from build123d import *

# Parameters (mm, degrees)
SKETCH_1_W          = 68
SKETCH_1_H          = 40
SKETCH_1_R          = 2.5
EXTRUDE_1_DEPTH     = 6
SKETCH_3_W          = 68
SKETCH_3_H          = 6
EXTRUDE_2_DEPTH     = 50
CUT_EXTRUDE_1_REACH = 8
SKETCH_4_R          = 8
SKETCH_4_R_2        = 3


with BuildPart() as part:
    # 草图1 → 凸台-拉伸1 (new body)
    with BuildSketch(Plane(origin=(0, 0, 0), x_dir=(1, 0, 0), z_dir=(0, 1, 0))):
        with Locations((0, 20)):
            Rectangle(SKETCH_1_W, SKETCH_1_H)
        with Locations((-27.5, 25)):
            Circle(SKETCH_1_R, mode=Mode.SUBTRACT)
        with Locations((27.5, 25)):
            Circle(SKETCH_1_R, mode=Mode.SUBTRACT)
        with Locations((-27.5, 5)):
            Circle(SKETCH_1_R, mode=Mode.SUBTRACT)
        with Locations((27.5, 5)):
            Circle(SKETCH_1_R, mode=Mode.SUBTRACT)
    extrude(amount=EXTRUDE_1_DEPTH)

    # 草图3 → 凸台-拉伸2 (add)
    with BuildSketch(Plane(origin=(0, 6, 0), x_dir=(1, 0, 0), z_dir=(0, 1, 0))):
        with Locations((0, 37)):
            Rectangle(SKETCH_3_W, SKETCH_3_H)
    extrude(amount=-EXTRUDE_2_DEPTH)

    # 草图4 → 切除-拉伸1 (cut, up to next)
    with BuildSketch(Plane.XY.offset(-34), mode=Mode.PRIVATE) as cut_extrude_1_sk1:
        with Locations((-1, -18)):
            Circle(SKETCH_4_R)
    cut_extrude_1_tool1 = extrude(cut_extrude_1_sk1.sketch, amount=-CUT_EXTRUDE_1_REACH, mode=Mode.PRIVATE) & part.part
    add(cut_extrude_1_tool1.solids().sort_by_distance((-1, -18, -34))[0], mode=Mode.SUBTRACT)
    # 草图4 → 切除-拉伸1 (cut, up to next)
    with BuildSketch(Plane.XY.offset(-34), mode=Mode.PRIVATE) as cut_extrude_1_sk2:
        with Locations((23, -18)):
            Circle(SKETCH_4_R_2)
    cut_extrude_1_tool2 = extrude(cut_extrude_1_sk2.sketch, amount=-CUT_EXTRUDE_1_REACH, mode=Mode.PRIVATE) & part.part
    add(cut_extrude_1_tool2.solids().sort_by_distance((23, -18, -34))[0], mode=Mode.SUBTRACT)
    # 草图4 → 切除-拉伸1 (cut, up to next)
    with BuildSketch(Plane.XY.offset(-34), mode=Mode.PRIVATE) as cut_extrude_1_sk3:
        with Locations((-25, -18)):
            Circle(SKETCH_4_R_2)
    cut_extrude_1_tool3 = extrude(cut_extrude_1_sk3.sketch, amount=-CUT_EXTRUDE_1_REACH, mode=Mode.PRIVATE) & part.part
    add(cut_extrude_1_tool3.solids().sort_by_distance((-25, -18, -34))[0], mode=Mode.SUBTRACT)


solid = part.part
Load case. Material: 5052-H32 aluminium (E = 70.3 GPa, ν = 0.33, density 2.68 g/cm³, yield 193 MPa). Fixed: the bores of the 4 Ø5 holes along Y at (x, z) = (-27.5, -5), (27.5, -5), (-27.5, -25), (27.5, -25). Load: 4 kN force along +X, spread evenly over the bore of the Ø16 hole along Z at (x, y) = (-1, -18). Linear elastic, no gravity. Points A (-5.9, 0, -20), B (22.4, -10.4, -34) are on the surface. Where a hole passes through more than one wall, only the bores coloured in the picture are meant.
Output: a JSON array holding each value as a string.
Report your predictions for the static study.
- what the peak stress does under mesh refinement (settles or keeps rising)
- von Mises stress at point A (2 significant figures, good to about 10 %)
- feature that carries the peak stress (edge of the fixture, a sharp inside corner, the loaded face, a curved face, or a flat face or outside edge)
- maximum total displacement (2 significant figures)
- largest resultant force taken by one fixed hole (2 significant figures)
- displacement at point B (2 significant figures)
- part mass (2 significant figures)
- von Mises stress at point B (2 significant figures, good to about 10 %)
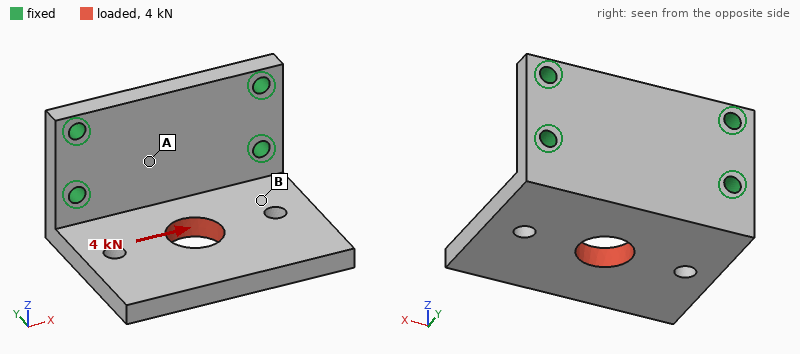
["keeps rising", "13 MPa", "edge of the fixture", "92 µm", "2.5 kN", "36 µm", "86 g", "35 MPa"]
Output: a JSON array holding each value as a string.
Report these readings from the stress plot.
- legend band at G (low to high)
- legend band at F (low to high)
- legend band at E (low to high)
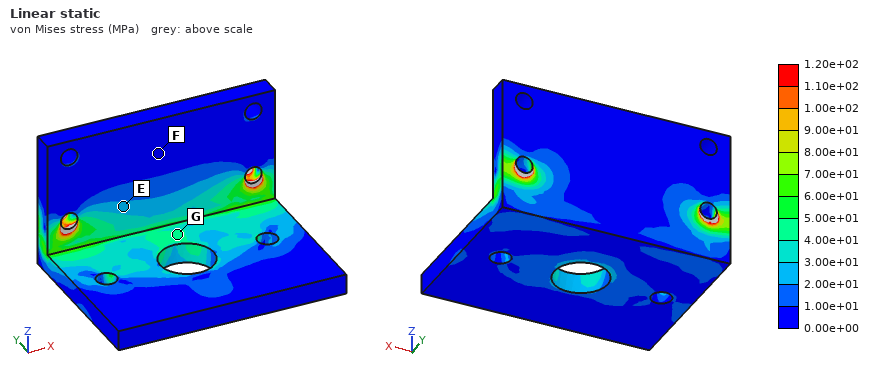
["4.00e+01 to 5.00e+01 MPa", "0.00e+00 to 1.00e+01 MPa", "2.00e+01 to 3.00e+01 MPa"]
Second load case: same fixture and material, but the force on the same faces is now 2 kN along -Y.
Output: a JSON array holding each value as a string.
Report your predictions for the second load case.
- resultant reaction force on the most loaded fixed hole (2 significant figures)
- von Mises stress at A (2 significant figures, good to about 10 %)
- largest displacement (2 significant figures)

["1.2 kN", "14 MPa", "0.11 mm"]
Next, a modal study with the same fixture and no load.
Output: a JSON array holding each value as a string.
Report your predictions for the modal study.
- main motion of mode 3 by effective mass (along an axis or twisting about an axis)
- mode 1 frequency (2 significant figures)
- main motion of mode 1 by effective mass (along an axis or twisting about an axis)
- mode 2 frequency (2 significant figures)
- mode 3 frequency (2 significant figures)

["along X", "1600 Hz", "along Z", "3300 Hz", "6100 Hz"]
